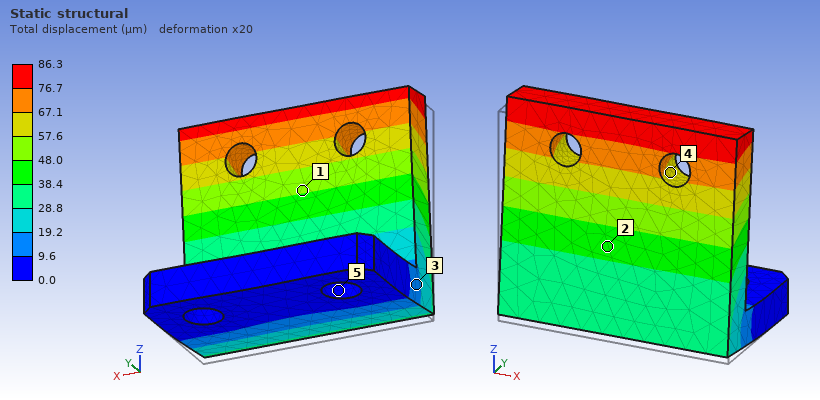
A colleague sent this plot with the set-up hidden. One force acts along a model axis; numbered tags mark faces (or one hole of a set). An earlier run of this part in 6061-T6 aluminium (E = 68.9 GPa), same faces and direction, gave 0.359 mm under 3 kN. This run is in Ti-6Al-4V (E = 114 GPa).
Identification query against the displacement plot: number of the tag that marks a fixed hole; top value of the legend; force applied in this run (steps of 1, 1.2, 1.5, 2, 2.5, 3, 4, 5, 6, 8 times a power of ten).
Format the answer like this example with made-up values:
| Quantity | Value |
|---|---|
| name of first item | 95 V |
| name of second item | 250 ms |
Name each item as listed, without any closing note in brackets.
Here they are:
| Quantity | Value |
|---|---|
| number of the tag that marks a fixed hole | 5 |
| top value of the legend | 86.3 µm |
| force applied in this run | 1.2 kN |
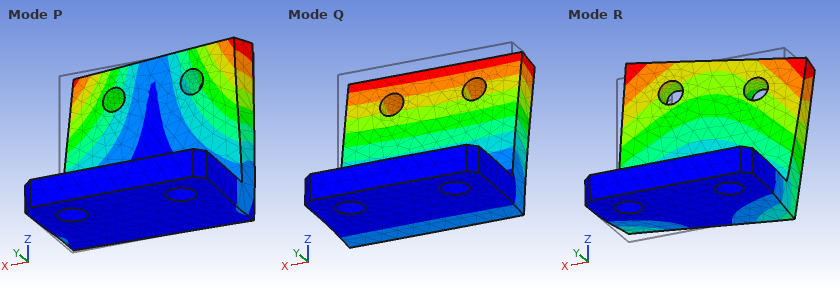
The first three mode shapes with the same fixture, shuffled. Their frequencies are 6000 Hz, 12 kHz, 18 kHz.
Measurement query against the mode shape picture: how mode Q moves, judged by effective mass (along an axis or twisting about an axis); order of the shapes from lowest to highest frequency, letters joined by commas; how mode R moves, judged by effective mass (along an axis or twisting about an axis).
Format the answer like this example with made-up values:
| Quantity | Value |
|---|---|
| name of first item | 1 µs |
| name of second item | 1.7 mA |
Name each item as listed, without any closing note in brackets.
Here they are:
| Quantity | Value |
|---|---|
| how mode Q moves, judged by effective mass | along Y |
| order of the shapes from lowest to highest frequency, letters joined by commas | Q, R, P |
| how mode R moves, judged by effective mass | along X |
